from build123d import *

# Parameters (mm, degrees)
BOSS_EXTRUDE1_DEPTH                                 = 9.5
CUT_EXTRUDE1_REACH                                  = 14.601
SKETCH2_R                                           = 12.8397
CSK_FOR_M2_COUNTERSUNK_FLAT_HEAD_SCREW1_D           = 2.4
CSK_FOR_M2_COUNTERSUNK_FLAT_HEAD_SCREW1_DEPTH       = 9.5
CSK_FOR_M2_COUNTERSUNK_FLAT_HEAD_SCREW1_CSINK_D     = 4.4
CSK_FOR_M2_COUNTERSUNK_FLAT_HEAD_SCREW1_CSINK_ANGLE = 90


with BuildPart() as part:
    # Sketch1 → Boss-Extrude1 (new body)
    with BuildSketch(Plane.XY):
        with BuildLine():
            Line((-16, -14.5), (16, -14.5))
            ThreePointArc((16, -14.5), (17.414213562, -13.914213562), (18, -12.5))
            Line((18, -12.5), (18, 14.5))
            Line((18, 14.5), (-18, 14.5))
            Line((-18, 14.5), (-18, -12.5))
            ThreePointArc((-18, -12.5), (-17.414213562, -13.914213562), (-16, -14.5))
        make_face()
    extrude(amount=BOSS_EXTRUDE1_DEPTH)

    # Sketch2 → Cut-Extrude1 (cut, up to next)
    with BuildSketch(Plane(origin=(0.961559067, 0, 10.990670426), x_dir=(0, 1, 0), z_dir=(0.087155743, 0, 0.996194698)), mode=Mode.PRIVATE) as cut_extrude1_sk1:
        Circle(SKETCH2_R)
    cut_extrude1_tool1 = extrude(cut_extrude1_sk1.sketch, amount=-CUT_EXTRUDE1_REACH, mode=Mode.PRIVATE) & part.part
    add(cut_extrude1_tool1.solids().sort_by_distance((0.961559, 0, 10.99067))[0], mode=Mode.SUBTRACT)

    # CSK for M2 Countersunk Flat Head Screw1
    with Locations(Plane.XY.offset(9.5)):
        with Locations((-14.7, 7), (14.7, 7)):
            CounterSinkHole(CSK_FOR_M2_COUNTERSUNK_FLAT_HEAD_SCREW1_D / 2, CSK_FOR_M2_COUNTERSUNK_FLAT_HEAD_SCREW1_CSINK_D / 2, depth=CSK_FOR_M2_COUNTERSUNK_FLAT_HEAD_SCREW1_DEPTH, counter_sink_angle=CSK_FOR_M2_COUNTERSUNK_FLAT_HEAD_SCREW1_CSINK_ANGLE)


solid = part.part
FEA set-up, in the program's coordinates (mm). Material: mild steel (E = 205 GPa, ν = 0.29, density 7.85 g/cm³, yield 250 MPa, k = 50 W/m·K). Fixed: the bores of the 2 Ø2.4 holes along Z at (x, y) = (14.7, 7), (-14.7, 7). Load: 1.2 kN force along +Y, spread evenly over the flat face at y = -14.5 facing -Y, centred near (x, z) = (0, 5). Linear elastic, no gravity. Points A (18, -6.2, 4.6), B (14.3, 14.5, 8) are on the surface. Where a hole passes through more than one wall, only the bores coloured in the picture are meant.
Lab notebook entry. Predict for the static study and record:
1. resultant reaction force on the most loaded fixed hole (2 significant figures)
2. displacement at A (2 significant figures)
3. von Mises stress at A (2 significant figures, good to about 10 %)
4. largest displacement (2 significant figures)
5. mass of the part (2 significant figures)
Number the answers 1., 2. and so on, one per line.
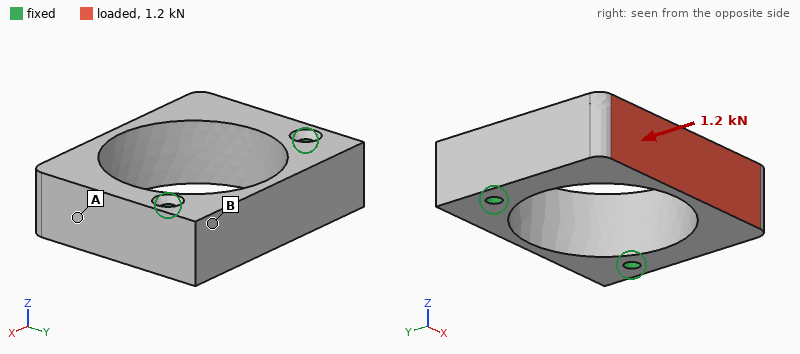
1. 700 N
2. 2.3 µm
3. 18 MPa
4. 8.1 µm
5. 38 g
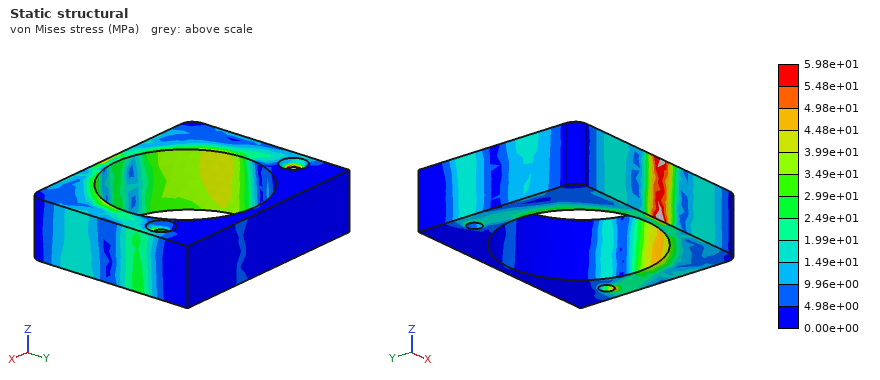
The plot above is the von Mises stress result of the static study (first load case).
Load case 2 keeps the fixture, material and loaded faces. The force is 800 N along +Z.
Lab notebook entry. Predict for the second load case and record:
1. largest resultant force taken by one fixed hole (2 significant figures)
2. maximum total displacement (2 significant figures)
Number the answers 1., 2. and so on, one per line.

1. 420 N
2. 27 µm
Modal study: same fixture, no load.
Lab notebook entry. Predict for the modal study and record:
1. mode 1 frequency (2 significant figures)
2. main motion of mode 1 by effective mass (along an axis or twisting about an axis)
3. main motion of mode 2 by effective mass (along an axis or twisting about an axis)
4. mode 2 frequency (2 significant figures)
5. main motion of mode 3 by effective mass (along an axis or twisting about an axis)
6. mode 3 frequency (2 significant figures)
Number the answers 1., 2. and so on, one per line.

1. 8900 Hz
2. along X
3. along Z
4. 9700 Hz
5. twisting about Y
6. 14 kHz
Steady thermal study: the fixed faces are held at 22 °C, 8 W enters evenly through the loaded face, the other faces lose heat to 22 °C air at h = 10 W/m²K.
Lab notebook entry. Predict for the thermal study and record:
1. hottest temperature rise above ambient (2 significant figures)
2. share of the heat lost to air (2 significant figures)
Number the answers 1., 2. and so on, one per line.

1. 36 K
2. 3.6 %
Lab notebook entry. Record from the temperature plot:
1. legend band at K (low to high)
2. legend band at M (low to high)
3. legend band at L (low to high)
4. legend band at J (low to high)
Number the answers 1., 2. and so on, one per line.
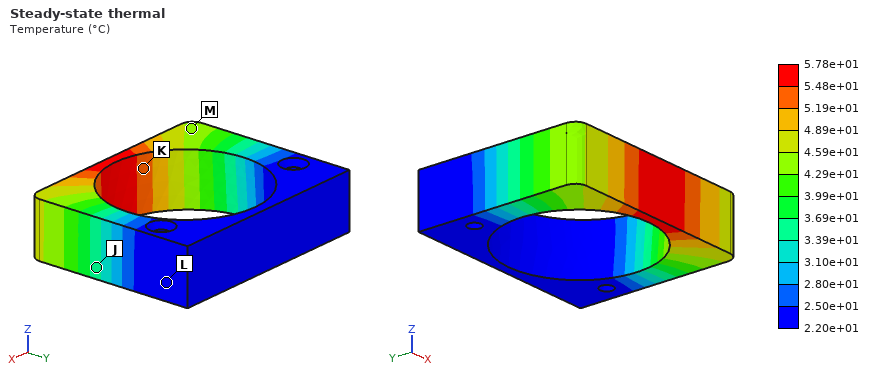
1. 5.19e+01 to 5.48e+01 °C
2. 4.29e+01 to 4.59e+01 °C
3. 2.20e+01 to 2.50e+01 °C
4. 3.39e+01 to 3.69e+01 °C
